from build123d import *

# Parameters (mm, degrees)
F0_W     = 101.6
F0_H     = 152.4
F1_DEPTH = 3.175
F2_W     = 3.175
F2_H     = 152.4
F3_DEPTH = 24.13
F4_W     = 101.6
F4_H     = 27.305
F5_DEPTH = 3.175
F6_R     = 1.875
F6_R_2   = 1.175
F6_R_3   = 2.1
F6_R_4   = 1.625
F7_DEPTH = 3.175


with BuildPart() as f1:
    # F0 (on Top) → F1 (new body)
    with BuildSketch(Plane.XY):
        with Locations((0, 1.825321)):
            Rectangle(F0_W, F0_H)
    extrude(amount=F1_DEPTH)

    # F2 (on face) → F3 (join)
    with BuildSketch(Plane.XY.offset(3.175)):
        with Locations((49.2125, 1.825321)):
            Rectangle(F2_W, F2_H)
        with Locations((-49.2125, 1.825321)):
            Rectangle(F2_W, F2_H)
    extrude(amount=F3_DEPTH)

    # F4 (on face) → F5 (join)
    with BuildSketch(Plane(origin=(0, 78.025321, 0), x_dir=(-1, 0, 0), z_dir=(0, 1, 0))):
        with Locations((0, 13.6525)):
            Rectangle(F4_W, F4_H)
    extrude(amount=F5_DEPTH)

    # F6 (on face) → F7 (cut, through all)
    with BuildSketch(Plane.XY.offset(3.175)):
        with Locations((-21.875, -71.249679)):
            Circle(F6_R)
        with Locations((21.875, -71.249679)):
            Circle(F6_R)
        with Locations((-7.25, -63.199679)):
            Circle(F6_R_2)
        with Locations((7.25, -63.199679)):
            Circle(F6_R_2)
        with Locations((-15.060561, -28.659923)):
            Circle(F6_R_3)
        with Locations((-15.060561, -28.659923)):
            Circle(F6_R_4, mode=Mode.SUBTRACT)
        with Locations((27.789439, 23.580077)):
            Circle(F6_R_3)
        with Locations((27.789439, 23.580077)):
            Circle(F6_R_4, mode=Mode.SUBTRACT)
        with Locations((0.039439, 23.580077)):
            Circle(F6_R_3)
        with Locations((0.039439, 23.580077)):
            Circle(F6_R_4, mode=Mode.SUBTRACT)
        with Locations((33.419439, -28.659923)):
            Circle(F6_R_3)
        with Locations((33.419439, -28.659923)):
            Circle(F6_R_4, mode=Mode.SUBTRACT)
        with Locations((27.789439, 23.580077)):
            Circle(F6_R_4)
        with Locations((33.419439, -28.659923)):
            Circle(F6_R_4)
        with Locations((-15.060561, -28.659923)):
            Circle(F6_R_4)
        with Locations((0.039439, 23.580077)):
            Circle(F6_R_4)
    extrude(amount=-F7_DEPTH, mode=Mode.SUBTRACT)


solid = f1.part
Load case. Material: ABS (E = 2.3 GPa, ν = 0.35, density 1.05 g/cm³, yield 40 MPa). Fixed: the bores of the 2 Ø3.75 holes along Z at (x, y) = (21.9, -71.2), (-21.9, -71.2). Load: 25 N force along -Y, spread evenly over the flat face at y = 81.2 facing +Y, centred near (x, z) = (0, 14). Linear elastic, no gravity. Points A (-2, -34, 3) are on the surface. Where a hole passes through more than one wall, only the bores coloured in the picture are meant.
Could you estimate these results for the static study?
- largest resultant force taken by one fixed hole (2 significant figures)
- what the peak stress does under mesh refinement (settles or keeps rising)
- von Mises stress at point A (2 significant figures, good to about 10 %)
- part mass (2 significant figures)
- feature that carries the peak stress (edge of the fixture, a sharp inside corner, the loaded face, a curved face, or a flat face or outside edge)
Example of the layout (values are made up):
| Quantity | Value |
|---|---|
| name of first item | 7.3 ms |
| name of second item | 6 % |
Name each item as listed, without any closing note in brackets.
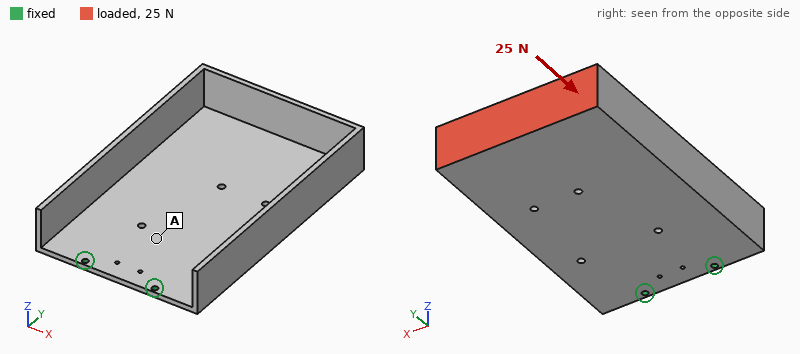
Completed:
| Quantity | Value |
|---|---|
| largest resultant force taken by one fixed hole | 13 N |
| what the peak stress does under mesh refinement | keeps rising |
| von Mises stress at point A | 0.45 MPa |
| part mass | 85 g |
| feature that carries the peak stress | edge of the fixture |
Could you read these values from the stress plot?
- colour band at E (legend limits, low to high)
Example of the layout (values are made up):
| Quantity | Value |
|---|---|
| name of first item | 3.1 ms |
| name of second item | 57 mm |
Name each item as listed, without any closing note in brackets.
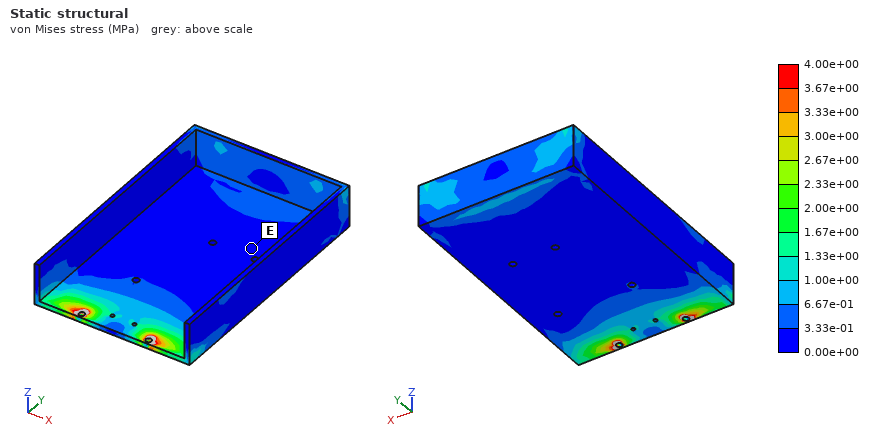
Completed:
| Quantity | Value |
|---|---|
| colour band at E | 0.00e+00 to 3.33e-01 MPa |
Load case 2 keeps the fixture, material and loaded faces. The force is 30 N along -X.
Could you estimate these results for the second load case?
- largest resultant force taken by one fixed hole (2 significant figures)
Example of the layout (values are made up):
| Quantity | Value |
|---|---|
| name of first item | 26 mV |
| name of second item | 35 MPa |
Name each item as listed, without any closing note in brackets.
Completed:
| Quantity | Value |
|---|---|
| largest resultant force taken by one fixed hole | 100 N |
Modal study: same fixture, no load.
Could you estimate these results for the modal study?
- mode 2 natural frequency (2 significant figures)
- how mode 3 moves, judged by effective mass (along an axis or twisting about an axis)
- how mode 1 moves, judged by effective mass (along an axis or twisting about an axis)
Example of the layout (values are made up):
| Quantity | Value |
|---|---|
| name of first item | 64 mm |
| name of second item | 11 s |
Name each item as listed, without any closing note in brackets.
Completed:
| Quantity | Value |
|---|---|
| mode 2 natural frequency | 73 Hz |
| how mode 3 moves, judged by effective mass | along Z |
| how mode 1 moves, judged by effective mass | along Z |
